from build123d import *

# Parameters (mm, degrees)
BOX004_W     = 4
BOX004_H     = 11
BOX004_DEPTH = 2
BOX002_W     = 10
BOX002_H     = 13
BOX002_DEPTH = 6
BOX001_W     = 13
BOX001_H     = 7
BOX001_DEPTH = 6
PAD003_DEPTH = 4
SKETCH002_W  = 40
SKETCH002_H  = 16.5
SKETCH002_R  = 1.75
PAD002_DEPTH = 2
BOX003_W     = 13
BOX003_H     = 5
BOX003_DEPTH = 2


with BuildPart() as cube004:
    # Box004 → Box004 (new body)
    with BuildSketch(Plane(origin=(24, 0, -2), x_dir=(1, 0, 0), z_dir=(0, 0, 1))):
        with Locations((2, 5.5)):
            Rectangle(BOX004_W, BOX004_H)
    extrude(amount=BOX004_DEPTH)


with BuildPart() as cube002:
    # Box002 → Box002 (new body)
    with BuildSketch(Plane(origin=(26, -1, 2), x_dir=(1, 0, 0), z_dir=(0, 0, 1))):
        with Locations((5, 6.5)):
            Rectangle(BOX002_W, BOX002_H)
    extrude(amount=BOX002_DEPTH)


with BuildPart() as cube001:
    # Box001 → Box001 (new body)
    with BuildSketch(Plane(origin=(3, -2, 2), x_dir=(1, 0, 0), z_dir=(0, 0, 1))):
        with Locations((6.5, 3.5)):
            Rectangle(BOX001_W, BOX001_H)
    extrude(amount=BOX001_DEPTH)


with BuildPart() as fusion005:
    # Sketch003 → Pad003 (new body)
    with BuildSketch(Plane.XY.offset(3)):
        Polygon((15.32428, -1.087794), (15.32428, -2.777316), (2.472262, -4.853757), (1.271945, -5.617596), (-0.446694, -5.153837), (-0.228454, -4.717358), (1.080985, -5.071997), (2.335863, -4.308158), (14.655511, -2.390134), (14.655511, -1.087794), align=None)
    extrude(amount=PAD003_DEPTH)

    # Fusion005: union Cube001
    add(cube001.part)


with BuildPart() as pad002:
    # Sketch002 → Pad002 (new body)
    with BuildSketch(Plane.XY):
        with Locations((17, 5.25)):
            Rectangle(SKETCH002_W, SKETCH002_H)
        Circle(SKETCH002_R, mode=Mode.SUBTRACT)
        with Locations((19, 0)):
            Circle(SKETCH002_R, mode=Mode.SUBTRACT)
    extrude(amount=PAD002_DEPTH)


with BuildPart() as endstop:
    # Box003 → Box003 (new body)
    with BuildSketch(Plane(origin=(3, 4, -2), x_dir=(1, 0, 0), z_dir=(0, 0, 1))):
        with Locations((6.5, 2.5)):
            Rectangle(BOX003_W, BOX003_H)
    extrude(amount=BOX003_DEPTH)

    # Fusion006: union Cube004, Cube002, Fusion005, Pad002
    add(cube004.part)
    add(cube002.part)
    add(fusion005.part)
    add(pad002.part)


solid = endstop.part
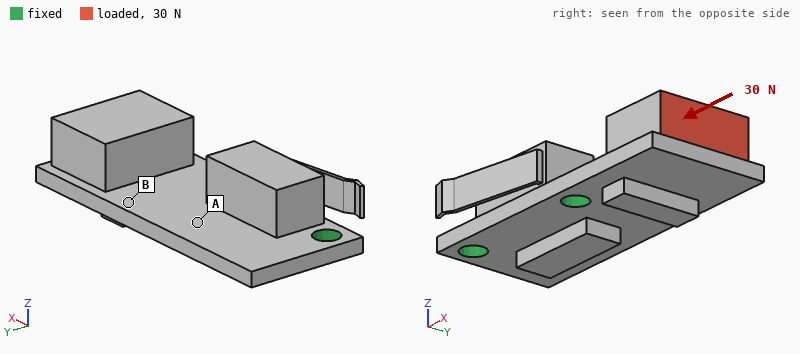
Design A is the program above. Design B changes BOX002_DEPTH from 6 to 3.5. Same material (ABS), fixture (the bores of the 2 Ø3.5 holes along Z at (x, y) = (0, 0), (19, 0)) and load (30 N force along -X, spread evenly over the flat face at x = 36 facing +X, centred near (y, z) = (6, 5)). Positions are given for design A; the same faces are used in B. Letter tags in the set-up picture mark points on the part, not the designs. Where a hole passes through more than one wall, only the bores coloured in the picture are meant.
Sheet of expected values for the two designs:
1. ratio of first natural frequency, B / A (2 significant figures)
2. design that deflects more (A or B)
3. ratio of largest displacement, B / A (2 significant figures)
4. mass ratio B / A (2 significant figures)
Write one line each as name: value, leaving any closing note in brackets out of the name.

ratio of first natural frequency, B / A: 1.00
design that deflects more: A
ratio of largest displacement, B / A: 0.68
mass ratio B / A: 0.89
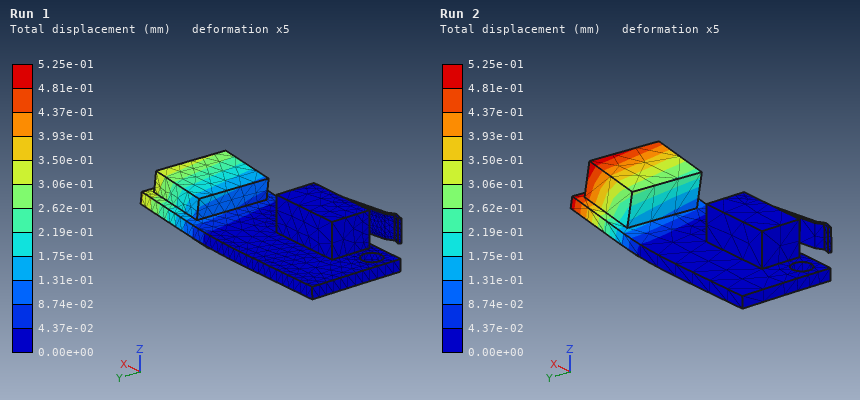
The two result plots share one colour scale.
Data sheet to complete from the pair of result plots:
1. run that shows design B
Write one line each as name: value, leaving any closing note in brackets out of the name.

run that shows design B: Run 1
